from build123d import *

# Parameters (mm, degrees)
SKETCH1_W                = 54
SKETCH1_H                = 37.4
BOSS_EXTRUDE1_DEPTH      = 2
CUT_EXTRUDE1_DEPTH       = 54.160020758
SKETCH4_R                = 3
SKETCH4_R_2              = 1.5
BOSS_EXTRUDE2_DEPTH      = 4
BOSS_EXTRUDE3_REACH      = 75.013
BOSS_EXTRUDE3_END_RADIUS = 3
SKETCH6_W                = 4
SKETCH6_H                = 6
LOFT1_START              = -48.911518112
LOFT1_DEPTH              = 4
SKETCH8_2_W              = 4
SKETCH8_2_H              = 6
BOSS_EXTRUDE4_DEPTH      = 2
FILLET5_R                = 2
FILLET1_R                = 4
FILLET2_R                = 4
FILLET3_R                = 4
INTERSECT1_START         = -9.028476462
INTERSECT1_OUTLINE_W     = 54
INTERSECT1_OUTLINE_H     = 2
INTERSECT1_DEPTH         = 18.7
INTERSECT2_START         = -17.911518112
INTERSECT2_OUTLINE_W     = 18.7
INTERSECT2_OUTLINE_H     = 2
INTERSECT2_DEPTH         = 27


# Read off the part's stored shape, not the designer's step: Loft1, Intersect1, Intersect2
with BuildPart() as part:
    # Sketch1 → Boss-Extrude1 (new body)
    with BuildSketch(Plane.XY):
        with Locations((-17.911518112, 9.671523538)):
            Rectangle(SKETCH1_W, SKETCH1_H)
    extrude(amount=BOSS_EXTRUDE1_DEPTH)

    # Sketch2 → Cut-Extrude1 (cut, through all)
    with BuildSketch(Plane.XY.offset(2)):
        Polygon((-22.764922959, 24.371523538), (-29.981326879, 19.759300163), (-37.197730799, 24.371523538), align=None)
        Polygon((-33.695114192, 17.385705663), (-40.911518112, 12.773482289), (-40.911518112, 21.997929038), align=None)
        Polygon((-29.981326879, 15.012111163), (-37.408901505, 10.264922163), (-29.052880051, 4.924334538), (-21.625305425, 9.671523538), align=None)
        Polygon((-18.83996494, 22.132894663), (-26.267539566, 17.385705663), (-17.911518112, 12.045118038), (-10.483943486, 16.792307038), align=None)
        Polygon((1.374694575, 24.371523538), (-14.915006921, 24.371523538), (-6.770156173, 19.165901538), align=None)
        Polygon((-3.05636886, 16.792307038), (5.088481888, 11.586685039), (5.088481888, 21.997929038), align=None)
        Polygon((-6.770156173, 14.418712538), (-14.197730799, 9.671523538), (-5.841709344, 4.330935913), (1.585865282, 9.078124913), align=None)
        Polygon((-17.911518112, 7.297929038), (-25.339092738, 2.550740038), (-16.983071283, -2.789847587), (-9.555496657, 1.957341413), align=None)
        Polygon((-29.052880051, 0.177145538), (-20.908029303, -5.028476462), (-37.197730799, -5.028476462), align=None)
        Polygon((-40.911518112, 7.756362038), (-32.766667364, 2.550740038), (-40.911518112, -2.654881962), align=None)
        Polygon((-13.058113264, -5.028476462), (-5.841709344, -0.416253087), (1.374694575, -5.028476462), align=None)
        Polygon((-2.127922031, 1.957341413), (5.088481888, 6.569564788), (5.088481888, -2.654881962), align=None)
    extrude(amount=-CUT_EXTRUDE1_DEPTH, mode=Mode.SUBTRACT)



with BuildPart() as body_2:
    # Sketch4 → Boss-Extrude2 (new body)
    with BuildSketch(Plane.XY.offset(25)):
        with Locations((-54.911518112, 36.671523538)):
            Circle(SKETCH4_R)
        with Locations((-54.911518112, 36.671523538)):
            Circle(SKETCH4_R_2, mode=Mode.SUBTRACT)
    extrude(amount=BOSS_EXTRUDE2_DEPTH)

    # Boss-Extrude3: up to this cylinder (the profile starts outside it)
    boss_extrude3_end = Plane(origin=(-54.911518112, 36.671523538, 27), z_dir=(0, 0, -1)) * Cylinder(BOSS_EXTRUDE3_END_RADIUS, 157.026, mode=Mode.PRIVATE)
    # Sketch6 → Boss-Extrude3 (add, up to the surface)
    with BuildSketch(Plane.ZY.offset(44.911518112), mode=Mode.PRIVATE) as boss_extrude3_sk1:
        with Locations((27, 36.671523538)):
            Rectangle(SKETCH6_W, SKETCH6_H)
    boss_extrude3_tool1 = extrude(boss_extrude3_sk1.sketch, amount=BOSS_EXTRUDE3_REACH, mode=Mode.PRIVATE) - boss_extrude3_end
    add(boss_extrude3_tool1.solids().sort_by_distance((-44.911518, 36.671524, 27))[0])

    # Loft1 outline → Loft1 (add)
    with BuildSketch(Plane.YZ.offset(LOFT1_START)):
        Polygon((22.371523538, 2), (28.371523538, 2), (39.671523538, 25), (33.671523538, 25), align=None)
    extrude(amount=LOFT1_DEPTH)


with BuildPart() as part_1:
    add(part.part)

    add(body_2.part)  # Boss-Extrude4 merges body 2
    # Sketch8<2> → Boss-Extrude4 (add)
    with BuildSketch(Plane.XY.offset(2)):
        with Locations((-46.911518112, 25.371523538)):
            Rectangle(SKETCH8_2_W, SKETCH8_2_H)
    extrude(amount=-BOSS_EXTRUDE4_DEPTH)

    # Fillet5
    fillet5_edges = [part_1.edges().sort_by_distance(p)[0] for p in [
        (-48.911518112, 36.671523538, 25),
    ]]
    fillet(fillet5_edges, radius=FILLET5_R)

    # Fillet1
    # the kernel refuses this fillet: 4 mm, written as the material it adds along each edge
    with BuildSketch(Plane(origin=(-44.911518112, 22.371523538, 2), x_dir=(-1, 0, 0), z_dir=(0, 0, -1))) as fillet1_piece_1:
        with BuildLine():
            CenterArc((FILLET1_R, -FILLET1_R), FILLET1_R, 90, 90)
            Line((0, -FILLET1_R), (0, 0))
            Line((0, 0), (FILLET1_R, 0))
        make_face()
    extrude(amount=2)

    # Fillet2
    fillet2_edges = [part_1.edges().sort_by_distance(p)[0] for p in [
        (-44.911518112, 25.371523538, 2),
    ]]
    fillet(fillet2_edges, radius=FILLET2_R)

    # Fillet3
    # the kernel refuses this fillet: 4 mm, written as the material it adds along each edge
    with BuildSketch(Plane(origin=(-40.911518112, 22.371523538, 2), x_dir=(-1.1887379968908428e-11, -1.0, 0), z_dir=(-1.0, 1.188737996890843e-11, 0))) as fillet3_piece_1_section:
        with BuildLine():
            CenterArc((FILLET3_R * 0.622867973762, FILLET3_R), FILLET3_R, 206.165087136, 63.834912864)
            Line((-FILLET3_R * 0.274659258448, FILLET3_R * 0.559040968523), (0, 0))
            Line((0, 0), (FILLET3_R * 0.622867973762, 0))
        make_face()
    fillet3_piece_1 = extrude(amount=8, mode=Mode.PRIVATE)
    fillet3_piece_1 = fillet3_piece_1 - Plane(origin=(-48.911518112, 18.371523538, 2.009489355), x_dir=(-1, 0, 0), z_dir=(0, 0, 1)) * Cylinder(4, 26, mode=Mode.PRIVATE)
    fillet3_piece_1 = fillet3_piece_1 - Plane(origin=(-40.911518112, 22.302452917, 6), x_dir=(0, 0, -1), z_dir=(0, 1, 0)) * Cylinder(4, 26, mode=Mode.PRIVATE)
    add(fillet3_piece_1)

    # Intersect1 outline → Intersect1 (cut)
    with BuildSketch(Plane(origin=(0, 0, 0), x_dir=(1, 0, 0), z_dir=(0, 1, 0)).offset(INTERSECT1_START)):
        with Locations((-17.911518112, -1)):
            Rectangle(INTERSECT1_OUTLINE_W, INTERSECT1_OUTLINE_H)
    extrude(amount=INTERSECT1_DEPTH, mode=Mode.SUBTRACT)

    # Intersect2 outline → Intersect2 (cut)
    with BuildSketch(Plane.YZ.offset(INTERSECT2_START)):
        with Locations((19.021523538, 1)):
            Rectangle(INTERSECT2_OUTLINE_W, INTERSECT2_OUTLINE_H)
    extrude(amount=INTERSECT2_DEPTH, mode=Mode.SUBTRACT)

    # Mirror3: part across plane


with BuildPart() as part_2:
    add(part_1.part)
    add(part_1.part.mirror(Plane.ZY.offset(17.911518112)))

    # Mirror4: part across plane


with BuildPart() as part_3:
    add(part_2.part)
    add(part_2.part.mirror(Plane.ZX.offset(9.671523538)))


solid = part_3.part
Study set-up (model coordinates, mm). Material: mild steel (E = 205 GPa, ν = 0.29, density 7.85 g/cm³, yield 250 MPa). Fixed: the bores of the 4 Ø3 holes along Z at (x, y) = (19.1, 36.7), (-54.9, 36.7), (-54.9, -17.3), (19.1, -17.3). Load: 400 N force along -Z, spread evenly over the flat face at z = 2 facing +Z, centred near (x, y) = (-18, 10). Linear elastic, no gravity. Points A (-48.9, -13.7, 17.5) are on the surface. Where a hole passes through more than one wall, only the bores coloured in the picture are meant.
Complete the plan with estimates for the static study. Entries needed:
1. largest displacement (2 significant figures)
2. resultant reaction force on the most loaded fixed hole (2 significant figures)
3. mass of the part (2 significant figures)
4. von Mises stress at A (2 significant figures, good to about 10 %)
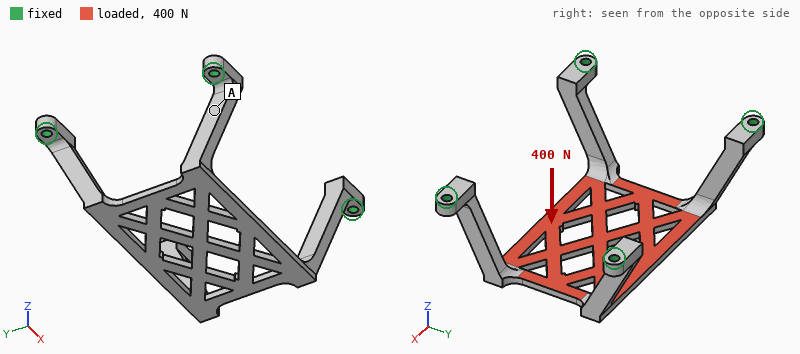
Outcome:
85 µm
130 N
50 g
12 MPa
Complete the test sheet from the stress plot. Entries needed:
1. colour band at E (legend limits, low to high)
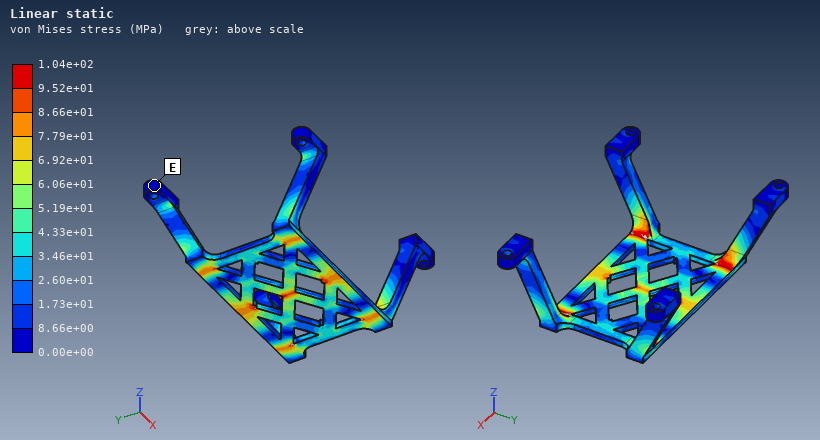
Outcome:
0.00e+00 to 8.66e+00 MPa
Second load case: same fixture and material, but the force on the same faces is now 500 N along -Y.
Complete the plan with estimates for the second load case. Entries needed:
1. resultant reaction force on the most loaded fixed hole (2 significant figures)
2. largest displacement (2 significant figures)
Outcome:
140 N
66 µm
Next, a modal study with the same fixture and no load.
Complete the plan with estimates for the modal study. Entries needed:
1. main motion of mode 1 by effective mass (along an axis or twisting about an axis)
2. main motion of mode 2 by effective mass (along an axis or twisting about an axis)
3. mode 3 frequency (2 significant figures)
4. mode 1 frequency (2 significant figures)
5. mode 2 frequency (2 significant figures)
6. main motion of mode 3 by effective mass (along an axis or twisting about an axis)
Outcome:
along X
along Y
2900 Hz
1900 Hz
2500 Hz
along Z
